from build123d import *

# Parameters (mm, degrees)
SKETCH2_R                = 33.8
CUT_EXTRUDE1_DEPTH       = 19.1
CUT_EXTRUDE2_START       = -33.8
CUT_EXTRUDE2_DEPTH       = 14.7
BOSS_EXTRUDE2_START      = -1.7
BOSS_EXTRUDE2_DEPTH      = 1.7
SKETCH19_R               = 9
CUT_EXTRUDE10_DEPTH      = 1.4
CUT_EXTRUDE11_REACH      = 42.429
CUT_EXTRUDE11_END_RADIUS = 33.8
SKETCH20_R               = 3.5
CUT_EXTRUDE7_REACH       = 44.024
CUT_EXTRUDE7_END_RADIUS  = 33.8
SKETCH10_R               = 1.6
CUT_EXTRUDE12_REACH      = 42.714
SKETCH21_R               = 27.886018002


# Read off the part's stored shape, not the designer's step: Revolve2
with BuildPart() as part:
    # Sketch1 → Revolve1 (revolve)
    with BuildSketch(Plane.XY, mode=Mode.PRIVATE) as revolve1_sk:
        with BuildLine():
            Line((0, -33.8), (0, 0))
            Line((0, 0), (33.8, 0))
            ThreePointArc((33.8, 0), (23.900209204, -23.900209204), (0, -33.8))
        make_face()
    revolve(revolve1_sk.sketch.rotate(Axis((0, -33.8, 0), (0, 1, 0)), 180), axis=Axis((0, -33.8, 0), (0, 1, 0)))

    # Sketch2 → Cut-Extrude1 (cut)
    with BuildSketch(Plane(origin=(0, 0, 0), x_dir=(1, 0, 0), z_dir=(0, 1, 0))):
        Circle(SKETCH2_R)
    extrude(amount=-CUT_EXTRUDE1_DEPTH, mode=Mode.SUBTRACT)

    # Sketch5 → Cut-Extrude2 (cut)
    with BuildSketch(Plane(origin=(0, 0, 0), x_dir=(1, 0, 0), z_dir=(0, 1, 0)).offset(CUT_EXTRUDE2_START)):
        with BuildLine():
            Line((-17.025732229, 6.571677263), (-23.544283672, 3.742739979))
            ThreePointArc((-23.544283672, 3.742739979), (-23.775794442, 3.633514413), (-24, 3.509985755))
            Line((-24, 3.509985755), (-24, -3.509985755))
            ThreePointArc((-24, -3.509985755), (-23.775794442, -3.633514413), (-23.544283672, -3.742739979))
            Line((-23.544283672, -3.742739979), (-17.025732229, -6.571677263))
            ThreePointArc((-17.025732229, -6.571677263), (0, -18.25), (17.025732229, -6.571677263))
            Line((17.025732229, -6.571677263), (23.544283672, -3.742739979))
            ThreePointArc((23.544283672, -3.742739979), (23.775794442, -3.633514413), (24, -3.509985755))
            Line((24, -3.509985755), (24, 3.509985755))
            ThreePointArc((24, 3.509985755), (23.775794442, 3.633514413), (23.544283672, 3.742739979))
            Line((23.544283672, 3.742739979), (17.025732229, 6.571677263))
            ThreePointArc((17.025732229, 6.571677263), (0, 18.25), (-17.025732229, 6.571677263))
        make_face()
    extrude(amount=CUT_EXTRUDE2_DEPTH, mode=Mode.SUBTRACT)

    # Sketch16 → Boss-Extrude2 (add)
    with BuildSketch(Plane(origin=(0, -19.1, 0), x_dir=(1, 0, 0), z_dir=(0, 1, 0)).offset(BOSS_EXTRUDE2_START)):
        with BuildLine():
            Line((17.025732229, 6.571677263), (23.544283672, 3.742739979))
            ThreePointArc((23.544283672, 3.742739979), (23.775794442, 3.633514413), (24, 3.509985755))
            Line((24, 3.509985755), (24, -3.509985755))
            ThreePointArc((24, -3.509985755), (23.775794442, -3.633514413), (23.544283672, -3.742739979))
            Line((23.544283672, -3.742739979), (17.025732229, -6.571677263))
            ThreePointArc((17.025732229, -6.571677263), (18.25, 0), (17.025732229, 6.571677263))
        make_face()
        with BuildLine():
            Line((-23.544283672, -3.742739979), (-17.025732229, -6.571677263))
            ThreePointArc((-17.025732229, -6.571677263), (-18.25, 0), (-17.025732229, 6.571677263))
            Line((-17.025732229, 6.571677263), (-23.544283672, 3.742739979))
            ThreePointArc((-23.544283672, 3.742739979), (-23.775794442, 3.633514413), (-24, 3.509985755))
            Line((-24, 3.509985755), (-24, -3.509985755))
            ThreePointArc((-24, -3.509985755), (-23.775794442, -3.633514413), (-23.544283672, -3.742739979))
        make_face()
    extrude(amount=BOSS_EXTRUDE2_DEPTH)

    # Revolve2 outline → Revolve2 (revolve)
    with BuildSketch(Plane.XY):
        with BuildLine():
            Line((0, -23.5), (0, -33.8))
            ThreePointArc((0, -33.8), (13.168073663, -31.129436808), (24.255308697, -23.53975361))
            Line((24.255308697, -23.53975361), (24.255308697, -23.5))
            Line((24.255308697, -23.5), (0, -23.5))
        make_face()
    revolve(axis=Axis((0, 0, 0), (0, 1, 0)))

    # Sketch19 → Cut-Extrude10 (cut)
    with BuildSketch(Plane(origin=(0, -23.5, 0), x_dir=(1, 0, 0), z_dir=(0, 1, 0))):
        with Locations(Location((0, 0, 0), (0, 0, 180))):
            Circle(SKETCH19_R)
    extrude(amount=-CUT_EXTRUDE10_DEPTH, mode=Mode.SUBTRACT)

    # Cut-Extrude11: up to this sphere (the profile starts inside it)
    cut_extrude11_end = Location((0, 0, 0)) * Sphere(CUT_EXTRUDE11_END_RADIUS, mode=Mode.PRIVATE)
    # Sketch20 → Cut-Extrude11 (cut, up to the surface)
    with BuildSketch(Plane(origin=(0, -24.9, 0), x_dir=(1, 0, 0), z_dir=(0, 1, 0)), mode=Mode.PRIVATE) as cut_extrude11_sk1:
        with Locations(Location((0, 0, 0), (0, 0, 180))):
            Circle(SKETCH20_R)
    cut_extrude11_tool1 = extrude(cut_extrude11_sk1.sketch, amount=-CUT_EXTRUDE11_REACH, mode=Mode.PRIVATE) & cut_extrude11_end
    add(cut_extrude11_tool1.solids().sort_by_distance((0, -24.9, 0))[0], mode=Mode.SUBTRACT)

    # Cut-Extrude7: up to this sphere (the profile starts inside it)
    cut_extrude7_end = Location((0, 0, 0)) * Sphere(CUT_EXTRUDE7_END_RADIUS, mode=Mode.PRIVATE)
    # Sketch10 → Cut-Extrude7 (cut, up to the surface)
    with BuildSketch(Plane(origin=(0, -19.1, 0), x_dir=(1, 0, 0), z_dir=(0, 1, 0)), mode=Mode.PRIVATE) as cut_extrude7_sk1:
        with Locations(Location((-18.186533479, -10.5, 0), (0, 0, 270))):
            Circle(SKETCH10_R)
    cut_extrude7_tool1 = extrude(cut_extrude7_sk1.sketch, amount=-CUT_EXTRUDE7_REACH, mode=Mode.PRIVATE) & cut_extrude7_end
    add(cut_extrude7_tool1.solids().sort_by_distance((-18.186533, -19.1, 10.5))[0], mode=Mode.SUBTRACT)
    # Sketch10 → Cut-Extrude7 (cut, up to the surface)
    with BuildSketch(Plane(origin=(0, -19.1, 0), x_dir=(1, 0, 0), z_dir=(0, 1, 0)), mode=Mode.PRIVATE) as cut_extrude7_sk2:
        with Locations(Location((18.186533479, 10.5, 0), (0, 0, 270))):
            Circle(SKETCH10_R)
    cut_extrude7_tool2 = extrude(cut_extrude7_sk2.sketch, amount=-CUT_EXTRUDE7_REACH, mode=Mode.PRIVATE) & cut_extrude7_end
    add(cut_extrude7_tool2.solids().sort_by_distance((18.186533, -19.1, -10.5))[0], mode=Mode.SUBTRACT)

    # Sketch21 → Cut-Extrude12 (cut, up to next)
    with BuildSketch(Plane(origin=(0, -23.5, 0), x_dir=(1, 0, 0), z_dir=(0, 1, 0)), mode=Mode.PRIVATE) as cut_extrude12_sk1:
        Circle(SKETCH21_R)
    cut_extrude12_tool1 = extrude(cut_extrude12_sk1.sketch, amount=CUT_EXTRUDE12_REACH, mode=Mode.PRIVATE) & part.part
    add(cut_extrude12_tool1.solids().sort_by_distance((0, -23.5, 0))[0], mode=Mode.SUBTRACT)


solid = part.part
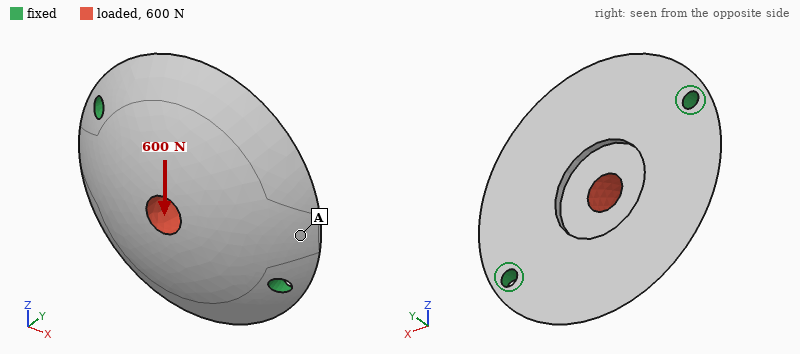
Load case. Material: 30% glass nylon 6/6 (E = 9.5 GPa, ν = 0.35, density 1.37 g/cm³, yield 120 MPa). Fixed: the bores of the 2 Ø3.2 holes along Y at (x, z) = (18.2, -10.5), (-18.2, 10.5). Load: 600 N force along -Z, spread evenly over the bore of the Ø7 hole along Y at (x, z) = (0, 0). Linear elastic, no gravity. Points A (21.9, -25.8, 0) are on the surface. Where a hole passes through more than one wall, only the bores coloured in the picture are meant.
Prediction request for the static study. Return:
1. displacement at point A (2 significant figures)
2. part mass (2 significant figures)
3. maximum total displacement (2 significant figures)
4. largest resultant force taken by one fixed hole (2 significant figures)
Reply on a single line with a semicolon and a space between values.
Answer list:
0.054 mm; 13 g; 0.14 mm; 300 N
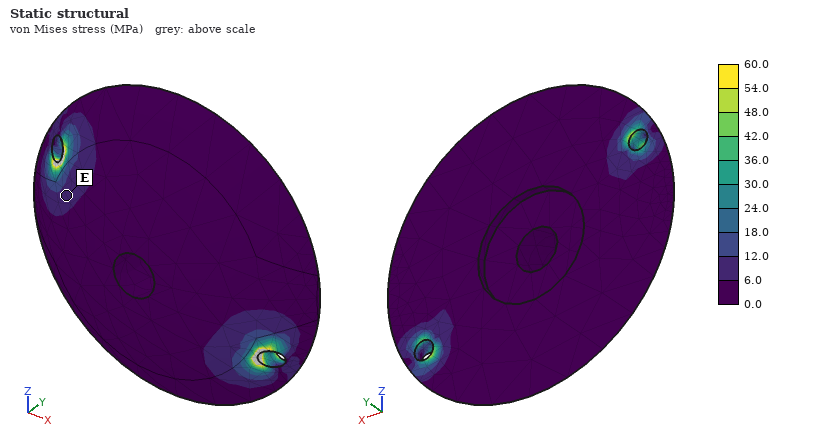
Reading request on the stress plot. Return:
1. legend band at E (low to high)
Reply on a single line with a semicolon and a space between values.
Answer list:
6.0 to 12.0 MPa
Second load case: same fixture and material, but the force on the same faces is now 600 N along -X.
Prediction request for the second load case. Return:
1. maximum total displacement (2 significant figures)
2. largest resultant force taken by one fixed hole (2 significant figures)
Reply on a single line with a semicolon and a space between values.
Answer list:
83 µm; 300 N
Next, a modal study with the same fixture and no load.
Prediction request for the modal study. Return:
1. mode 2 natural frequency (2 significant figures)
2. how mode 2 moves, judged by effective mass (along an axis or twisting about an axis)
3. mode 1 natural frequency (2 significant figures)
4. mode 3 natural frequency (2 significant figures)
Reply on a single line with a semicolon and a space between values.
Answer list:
4900 Hz; along Y; 2400 Hz; 10 kHz
